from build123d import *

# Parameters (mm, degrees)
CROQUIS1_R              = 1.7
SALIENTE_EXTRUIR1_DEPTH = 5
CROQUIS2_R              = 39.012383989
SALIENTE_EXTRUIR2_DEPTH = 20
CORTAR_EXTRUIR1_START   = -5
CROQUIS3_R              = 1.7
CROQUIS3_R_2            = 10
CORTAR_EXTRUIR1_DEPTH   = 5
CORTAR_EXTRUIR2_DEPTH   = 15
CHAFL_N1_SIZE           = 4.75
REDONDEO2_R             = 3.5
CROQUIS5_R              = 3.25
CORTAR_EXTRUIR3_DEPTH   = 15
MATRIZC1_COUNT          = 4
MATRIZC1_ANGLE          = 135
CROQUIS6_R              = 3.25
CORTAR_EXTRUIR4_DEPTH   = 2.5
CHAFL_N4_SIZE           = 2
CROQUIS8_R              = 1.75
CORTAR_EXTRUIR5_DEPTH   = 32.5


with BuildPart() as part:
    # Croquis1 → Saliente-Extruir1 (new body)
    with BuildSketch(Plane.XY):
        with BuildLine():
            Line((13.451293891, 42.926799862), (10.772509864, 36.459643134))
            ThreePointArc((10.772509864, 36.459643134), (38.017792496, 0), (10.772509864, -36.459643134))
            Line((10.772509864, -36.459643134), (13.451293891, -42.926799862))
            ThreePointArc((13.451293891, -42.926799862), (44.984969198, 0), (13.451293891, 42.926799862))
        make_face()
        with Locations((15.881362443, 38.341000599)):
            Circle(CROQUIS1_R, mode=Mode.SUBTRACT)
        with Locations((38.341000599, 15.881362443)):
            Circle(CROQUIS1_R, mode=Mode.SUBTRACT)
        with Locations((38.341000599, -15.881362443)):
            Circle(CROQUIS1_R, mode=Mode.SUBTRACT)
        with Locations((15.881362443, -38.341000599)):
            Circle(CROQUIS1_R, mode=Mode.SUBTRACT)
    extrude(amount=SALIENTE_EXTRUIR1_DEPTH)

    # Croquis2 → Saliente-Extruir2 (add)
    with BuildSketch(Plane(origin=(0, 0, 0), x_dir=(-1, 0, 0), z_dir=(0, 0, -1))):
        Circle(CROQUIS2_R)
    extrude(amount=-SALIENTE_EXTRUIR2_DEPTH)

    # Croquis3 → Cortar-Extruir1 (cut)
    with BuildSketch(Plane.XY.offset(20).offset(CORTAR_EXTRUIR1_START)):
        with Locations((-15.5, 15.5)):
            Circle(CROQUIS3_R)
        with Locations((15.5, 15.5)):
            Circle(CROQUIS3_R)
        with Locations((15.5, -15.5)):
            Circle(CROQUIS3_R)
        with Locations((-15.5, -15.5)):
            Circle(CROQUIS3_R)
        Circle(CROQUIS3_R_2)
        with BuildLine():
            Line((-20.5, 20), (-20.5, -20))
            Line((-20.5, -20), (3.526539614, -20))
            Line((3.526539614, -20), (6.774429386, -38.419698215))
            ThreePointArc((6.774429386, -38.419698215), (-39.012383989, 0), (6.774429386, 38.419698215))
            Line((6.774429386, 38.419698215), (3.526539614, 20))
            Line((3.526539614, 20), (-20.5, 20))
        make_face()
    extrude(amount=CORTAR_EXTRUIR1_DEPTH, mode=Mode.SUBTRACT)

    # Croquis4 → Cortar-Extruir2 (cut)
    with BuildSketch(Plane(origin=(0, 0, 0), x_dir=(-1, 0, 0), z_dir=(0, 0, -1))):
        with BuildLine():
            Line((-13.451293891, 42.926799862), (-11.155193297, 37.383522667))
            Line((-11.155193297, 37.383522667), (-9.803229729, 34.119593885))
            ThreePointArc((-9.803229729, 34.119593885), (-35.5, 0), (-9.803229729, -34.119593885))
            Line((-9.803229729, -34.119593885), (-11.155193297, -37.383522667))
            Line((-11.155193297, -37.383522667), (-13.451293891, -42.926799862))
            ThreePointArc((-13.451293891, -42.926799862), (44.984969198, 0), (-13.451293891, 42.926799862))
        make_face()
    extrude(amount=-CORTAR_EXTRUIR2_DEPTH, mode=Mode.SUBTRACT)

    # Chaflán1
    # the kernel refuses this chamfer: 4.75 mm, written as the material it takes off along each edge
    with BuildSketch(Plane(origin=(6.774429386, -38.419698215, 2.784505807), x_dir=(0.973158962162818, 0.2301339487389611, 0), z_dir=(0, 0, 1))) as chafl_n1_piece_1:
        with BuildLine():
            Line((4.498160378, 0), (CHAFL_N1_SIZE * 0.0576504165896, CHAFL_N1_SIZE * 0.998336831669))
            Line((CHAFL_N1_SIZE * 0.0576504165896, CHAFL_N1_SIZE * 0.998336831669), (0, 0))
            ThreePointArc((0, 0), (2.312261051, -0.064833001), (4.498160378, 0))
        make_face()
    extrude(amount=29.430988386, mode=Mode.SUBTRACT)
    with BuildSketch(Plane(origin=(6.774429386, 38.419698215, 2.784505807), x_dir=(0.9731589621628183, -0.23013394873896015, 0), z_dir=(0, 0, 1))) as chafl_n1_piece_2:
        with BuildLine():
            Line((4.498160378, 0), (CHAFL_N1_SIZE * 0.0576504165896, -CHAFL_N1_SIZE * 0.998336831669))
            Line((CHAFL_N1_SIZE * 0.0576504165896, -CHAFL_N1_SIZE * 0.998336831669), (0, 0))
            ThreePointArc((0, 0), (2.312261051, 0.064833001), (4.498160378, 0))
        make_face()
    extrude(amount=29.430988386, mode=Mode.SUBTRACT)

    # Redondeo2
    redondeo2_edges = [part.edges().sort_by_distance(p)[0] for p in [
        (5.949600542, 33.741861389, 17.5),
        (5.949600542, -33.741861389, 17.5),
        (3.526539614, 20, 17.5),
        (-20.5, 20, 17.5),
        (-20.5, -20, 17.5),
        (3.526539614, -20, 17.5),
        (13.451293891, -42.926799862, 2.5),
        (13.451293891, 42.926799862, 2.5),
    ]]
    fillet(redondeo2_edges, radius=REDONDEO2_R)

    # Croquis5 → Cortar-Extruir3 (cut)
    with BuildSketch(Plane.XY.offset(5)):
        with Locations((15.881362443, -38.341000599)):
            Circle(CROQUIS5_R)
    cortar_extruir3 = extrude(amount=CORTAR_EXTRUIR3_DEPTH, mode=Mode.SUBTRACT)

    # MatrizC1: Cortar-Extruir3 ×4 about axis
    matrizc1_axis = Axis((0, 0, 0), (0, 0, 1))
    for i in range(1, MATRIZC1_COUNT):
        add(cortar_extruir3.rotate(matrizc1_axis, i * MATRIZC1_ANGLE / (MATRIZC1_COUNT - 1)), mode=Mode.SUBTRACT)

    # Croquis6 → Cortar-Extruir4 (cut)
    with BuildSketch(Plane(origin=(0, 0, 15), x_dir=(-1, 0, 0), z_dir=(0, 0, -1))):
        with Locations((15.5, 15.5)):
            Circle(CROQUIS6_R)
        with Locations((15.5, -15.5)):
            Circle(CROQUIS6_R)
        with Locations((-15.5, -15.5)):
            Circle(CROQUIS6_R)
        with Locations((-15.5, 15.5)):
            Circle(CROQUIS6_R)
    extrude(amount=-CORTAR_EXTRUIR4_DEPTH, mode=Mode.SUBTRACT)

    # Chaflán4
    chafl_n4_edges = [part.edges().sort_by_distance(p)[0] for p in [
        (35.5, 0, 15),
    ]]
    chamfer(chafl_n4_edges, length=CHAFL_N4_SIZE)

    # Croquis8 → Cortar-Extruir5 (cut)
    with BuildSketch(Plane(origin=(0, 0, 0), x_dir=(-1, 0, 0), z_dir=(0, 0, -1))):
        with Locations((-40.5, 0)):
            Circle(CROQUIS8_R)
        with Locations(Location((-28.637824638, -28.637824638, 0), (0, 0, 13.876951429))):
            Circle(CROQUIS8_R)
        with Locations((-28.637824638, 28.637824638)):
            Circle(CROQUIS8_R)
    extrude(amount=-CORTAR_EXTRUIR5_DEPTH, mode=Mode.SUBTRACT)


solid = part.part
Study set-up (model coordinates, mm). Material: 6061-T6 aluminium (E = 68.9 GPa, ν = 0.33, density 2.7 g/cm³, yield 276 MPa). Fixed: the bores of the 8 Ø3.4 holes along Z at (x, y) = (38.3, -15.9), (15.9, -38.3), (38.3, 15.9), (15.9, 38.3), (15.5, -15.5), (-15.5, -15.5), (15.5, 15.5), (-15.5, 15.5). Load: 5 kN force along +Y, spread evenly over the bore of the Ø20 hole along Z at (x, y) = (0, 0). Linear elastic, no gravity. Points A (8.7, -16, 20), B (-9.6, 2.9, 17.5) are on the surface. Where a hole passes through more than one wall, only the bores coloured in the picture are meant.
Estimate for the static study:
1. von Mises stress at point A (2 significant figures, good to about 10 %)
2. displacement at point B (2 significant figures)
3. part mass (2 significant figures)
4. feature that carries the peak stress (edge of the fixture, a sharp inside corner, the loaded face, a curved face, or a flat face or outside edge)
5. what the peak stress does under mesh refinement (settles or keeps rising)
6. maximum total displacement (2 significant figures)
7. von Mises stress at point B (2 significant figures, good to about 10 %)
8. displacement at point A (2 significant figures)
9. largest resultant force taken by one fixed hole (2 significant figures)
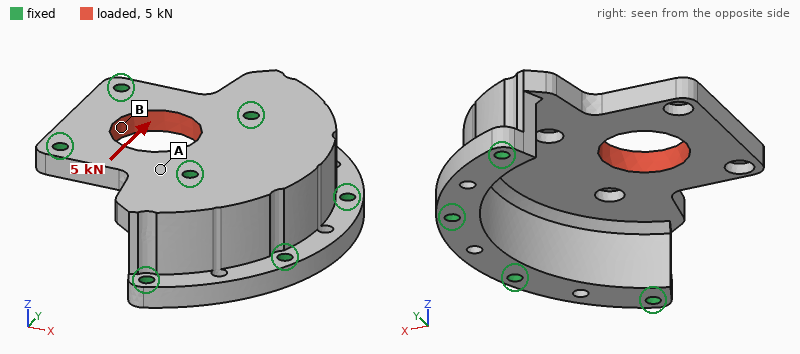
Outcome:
12 MPa
6.4 µm
56 g
edge of the fixture
keeps rising
10 µm
32 MPa
4.5 µm
1.4 kN
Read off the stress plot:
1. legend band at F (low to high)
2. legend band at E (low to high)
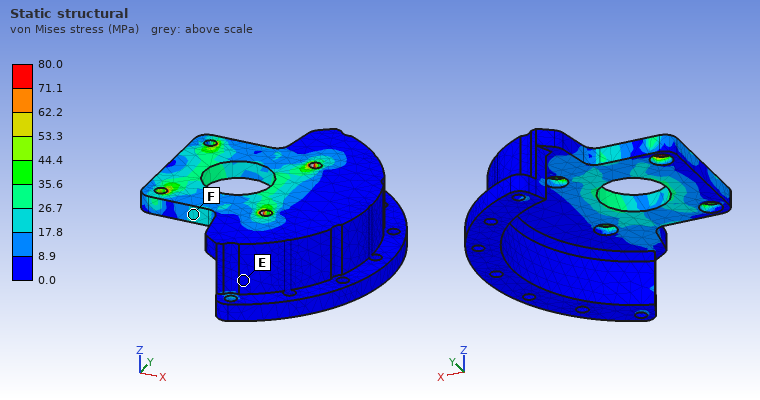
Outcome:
17.8 to 26.7 MPa
0.0 to 8.9 MPa
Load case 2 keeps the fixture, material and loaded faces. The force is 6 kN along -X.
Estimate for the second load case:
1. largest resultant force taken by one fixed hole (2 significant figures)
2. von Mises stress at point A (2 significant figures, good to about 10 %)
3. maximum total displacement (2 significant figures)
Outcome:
1.6 kN
29 MPa
15 µm
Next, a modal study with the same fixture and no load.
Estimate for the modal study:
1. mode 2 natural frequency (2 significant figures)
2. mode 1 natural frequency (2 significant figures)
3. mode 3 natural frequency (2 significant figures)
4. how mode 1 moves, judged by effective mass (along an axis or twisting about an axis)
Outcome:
20 kHz
17 kHz
21 kHz
along Z
